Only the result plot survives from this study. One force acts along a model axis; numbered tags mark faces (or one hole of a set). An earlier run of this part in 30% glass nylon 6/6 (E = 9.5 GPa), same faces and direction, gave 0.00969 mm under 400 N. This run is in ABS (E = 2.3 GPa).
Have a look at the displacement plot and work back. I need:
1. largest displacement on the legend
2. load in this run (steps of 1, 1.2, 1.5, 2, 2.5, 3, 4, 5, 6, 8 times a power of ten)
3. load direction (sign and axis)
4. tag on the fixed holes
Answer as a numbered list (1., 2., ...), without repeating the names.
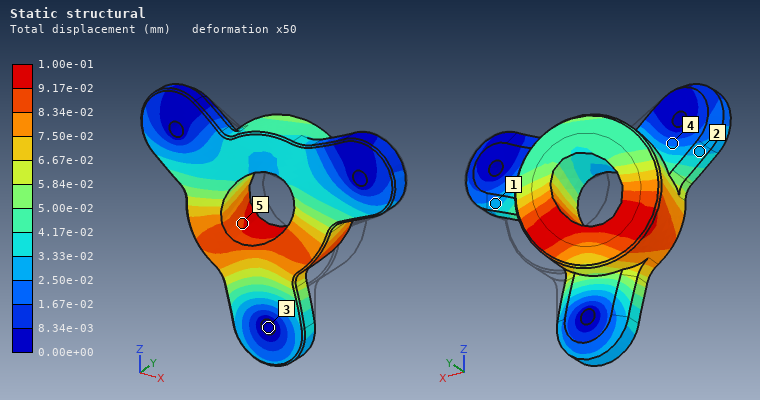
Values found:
1. 1.00e-01 mm
2. 1 kN
3. -X
4. 3
